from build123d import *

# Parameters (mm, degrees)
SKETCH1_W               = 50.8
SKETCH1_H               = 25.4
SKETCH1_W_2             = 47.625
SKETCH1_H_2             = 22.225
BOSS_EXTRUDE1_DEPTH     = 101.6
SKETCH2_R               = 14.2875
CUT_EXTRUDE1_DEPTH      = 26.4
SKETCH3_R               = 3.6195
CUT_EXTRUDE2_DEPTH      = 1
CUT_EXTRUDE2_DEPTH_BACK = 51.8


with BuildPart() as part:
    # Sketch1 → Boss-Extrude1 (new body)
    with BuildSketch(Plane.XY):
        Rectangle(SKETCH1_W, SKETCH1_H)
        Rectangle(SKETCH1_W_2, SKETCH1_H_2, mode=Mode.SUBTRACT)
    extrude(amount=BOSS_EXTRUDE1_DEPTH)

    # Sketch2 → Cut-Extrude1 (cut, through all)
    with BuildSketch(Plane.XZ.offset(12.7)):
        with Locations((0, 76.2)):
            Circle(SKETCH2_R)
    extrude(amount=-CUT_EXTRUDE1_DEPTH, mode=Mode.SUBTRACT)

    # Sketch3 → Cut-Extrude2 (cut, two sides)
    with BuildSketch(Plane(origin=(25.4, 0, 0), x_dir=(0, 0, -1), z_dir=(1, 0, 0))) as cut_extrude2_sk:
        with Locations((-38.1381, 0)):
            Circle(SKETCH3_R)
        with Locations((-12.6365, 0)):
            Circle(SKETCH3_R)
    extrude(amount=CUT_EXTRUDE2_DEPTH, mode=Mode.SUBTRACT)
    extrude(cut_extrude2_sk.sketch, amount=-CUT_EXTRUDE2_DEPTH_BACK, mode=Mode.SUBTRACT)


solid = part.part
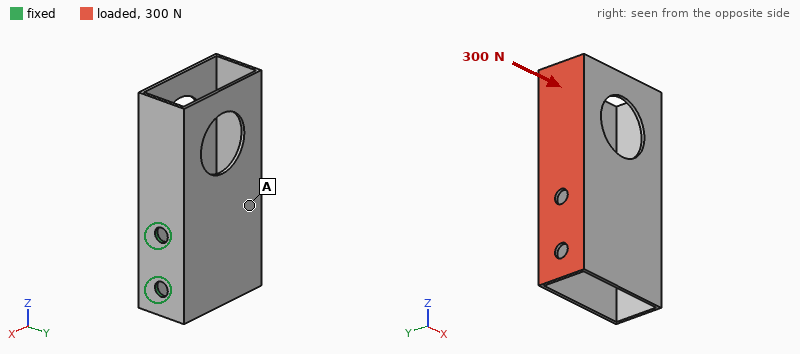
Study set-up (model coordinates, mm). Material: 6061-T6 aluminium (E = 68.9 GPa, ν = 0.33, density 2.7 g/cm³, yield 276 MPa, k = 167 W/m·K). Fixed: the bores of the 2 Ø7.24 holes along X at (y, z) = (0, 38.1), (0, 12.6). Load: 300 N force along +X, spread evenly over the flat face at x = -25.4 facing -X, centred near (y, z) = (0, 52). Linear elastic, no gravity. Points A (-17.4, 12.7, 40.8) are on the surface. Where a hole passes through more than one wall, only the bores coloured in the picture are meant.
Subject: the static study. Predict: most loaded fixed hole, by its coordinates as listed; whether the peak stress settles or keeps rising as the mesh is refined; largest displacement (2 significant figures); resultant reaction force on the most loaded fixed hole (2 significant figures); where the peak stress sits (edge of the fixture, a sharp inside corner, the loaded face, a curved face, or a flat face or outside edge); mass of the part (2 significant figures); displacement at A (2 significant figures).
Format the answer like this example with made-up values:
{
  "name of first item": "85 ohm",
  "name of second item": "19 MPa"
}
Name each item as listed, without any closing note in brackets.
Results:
{
  "most loaded fixed hole, by its coordinates as listed": "(0, 38.1)",
  "whether the peak stress settles or keeps rising as the mesh is refined": "keeps rising",
  "largest displacement": "0.27 mm",
  "resultant reaction force on the most loaded fixed hole": "400 N",
  "where the peak stress sits": "edge of the fixture",
  "mass of the part": "57 g",
  "displacement at A": "0.12 mm"
}
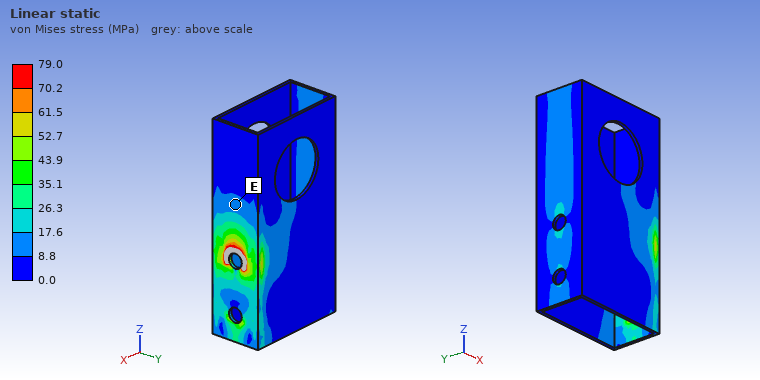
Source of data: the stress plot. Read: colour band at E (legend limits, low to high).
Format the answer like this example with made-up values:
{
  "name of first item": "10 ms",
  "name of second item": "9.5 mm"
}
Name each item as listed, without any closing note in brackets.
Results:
{
  "colour band at E": "8.8 to 17.6 MPa"
}
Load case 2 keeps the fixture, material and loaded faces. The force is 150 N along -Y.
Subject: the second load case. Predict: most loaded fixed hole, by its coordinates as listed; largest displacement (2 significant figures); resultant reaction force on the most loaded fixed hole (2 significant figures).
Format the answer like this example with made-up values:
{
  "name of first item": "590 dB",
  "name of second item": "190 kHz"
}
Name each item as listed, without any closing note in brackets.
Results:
{
  "most loaded fixed hole, by its coordinates as listed": "(0, 38.1)",
  "largest displacement": "1.1 mm",
  "resultant reaction force on the most loaded fixed hole": "180 N"
}
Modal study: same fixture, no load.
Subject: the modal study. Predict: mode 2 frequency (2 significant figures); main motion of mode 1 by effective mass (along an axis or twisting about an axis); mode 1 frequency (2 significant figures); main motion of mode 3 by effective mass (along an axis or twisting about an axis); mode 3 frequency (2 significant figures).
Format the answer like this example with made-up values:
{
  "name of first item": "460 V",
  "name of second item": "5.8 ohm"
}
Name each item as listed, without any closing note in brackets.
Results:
{
  "mode 2 frequency": "740 Hz",
  "main motion of mode 1 by effective mass": "along Y",
  "mode 1 frequency": "390 Hz",
  "main motion of mode 3 by effective mass": "twisting about X",
  "mode 3 frequency": "1200 Hz"
}
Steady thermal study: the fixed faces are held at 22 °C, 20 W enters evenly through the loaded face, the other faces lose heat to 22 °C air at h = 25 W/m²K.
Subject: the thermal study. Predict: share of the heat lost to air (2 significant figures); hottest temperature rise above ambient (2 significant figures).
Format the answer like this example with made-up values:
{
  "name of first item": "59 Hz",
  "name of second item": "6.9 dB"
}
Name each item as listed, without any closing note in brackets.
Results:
{
  "share of the heat lost to air": "45 %",
  "hottest temperature rise above ambient": "29 K"
}
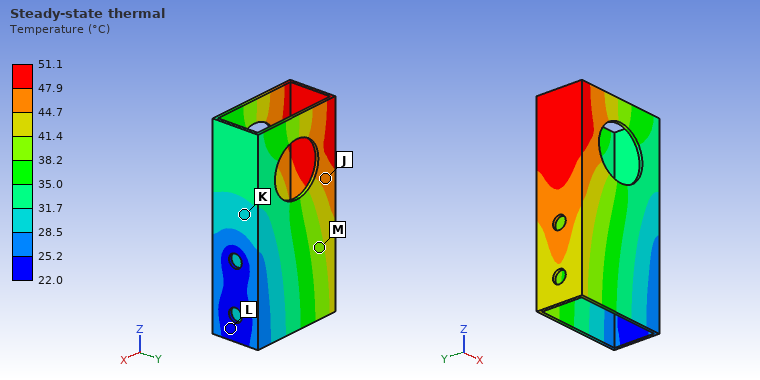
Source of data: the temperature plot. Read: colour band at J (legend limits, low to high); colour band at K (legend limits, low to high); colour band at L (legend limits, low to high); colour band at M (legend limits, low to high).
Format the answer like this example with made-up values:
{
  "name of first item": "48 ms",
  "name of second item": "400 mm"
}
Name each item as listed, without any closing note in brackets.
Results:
{
  "colour band at J": "44.7 to 47.9 °C",
  "colour band at K": "28.5 to 31.7 °C",
  "colour band at L": "22.0 to 25.2 °C",
  "colour band at M": "38.2 to 41.4 °C"
}
